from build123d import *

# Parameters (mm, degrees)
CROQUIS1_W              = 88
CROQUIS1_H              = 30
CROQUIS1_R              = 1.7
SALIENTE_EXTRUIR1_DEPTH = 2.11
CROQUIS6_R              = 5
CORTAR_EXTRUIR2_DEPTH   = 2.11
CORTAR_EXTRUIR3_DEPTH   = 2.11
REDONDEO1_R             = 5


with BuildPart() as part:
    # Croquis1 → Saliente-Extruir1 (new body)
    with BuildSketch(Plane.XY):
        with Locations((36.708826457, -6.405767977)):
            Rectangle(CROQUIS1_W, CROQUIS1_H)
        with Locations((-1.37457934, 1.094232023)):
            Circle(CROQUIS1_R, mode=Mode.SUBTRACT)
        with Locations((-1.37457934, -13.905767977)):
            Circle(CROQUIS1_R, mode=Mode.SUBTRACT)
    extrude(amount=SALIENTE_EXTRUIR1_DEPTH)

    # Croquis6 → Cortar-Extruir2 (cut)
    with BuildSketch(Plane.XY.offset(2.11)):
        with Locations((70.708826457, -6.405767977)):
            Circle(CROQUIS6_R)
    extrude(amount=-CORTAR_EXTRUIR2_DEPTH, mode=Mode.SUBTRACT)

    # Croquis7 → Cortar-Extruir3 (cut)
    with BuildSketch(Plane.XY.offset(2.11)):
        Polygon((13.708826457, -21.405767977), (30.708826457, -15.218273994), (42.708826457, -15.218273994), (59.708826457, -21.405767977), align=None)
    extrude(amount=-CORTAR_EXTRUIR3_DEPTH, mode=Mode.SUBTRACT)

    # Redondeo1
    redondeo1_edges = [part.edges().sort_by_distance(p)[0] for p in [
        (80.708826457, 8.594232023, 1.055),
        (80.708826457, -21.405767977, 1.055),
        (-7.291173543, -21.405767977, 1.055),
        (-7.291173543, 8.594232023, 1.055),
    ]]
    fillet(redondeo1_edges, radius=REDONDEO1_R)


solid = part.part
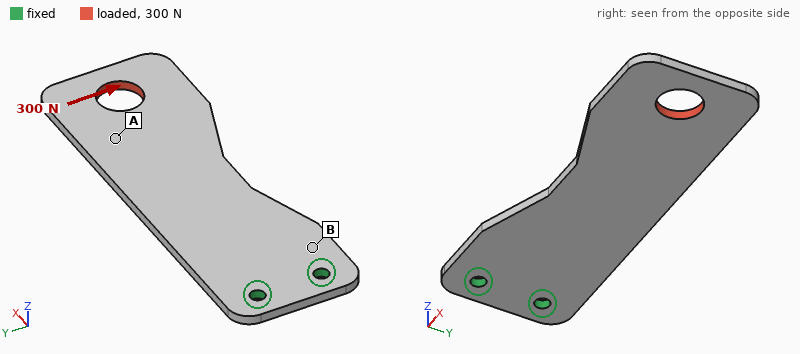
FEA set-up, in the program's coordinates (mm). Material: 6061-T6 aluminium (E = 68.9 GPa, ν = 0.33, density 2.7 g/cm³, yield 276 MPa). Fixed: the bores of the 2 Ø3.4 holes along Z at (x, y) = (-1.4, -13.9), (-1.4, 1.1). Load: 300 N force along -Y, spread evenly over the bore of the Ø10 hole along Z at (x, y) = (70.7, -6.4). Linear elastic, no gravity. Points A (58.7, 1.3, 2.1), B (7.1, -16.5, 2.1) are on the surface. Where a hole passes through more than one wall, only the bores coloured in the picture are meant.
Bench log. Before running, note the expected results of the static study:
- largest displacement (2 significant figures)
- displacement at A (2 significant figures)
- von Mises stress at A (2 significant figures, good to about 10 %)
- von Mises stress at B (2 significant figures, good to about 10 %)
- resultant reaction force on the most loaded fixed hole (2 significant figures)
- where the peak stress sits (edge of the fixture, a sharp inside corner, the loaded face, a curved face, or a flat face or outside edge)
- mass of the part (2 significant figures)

0.24 mm
0.15 mm
12 MPa
46 MPa
1.3 kN
edge of the fixture
13 g
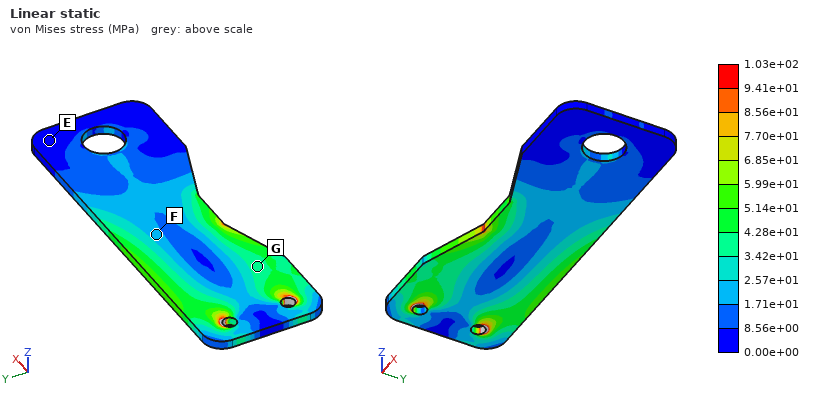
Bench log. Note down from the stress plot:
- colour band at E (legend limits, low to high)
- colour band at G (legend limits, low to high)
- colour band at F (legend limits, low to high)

0.00e+00 to 8.56e+00 MPa
3.42e+01 to 4.28e+01 MPa
1.71e+01 to 2.57e+01 MPa
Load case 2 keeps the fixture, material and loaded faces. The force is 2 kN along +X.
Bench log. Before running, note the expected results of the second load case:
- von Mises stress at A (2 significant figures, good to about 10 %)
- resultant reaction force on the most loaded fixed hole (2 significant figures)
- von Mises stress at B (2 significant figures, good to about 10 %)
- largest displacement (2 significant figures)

36 MPa
1.0 kN
34 MPa
73 µm
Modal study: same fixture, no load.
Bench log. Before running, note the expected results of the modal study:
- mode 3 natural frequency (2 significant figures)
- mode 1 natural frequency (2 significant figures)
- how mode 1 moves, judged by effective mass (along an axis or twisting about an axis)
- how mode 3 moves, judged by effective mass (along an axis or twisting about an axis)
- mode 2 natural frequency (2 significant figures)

1700 Hz
270 Hz
along Z
along Z
1400 Hz
